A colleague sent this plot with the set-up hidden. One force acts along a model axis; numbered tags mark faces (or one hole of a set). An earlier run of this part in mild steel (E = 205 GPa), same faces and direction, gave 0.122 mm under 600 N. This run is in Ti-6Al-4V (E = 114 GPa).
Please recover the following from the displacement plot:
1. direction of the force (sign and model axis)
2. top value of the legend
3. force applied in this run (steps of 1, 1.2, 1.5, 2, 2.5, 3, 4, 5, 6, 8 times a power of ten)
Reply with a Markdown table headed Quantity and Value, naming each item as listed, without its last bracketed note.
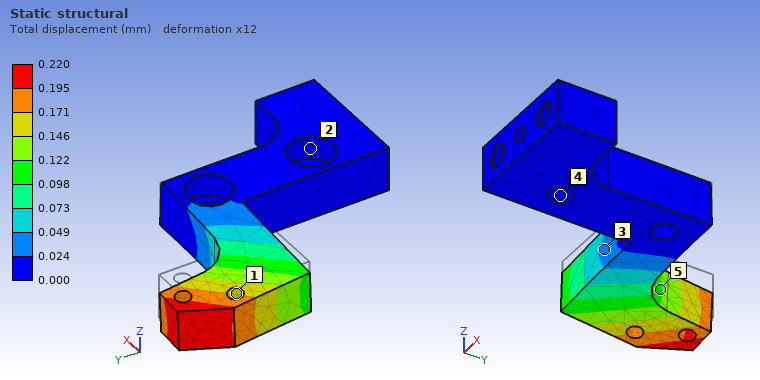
| Quantity | Value |
|---|---|
| direction of the force | -Z |
| top value of the legend | 0.220 mm |
| force applied in this run | 600 N |
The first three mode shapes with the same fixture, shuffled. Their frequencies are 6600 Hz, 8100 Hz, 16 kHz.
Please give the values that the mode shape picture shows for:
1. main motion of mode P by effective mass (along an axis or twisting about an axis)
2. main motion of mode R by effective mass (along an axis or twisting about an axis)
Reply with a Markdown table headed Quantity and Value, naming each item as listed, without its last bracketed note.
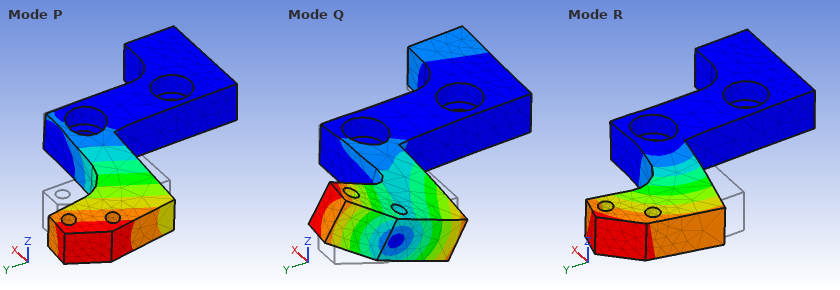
| Quantity | Value |
|---|---|
| main motion of mode P by effective mass | along Z |
| main motion of mode R by effective mass | along Y |
